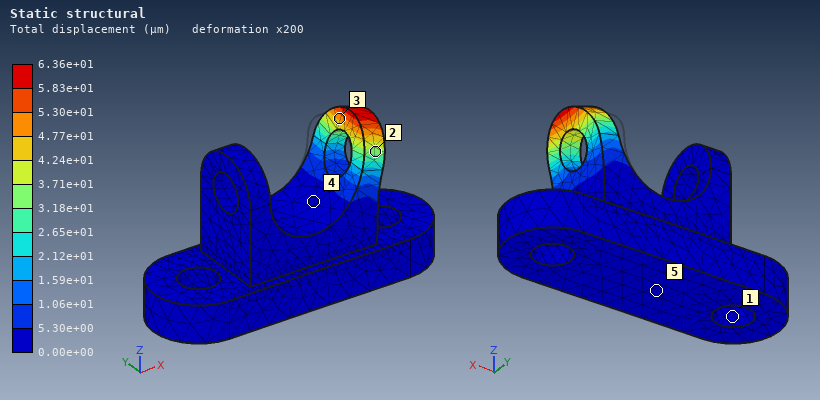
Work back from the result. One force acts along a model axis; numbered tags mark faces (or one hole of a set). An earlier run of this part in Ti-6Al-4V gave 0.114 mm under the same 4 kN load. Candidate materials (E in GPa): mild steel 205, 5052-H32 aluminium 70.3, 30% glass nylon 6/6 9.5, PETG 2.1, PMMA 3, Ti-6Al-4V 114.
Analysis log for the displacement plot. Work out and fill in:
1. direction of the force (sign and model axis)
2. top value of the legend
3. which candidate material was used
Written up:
+X
6.36e+01 µm
mild steel
